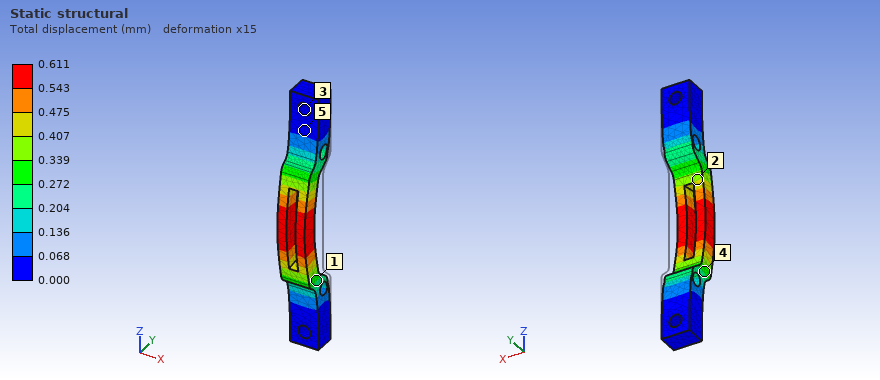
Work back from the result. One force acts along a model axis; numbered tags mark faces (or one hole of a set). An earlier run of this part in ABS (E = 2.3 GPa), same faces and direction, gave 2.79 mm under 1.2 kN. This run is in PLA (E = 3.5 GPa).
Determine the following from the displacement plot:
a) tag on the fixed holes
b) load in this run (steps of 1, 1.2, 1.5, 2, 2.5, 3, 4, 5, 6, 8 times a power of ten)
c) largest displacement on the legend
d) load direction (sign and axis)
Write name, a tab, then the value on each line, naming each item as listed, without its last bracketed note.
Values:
tag on the fixed holes	3
load in this run	400 N
largest displacement on the legend	0.611 mm
load direction	-Y
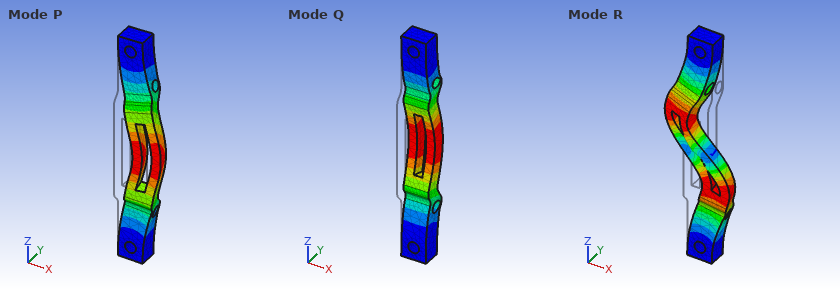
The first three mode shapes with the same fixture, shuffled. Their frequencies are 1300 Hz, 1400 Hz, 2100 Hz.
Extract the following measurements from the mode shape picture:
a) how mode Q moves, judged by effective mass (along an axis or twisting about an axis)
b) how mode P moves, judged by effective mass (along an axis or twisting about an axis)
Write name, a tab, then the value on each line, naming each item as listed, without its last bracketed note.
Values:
how mode Q moves, judged by effective mass	along Y
how mode P moves, judged by effective mass	along X
